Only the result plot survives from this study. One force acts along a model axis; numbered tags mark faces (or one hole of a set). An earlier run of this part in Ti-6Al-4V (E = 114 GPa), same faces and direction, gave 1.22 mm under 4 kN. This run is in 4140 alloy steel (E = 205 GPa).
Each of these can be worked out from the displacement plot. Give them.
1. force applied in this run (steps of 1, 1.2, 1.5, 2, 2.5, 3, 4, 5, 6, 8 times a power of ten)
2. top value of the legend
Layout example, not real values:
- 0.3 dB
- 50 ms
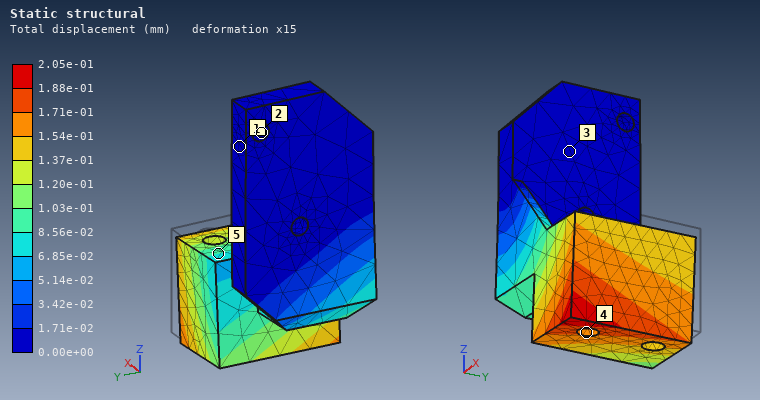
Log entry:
- 1.2 kN
- 2.05e-01 mm
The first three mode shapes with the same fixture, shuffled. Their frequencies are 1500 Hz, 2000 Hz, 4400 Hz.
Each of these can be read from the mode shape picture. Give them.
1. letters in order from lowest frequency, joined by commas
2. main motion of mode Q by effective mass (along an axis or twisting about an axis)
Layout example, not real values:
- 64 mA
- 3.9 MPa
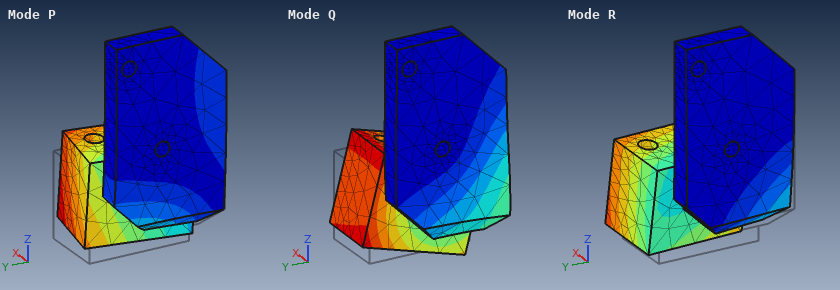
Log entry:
- R, P, Q
- along X
